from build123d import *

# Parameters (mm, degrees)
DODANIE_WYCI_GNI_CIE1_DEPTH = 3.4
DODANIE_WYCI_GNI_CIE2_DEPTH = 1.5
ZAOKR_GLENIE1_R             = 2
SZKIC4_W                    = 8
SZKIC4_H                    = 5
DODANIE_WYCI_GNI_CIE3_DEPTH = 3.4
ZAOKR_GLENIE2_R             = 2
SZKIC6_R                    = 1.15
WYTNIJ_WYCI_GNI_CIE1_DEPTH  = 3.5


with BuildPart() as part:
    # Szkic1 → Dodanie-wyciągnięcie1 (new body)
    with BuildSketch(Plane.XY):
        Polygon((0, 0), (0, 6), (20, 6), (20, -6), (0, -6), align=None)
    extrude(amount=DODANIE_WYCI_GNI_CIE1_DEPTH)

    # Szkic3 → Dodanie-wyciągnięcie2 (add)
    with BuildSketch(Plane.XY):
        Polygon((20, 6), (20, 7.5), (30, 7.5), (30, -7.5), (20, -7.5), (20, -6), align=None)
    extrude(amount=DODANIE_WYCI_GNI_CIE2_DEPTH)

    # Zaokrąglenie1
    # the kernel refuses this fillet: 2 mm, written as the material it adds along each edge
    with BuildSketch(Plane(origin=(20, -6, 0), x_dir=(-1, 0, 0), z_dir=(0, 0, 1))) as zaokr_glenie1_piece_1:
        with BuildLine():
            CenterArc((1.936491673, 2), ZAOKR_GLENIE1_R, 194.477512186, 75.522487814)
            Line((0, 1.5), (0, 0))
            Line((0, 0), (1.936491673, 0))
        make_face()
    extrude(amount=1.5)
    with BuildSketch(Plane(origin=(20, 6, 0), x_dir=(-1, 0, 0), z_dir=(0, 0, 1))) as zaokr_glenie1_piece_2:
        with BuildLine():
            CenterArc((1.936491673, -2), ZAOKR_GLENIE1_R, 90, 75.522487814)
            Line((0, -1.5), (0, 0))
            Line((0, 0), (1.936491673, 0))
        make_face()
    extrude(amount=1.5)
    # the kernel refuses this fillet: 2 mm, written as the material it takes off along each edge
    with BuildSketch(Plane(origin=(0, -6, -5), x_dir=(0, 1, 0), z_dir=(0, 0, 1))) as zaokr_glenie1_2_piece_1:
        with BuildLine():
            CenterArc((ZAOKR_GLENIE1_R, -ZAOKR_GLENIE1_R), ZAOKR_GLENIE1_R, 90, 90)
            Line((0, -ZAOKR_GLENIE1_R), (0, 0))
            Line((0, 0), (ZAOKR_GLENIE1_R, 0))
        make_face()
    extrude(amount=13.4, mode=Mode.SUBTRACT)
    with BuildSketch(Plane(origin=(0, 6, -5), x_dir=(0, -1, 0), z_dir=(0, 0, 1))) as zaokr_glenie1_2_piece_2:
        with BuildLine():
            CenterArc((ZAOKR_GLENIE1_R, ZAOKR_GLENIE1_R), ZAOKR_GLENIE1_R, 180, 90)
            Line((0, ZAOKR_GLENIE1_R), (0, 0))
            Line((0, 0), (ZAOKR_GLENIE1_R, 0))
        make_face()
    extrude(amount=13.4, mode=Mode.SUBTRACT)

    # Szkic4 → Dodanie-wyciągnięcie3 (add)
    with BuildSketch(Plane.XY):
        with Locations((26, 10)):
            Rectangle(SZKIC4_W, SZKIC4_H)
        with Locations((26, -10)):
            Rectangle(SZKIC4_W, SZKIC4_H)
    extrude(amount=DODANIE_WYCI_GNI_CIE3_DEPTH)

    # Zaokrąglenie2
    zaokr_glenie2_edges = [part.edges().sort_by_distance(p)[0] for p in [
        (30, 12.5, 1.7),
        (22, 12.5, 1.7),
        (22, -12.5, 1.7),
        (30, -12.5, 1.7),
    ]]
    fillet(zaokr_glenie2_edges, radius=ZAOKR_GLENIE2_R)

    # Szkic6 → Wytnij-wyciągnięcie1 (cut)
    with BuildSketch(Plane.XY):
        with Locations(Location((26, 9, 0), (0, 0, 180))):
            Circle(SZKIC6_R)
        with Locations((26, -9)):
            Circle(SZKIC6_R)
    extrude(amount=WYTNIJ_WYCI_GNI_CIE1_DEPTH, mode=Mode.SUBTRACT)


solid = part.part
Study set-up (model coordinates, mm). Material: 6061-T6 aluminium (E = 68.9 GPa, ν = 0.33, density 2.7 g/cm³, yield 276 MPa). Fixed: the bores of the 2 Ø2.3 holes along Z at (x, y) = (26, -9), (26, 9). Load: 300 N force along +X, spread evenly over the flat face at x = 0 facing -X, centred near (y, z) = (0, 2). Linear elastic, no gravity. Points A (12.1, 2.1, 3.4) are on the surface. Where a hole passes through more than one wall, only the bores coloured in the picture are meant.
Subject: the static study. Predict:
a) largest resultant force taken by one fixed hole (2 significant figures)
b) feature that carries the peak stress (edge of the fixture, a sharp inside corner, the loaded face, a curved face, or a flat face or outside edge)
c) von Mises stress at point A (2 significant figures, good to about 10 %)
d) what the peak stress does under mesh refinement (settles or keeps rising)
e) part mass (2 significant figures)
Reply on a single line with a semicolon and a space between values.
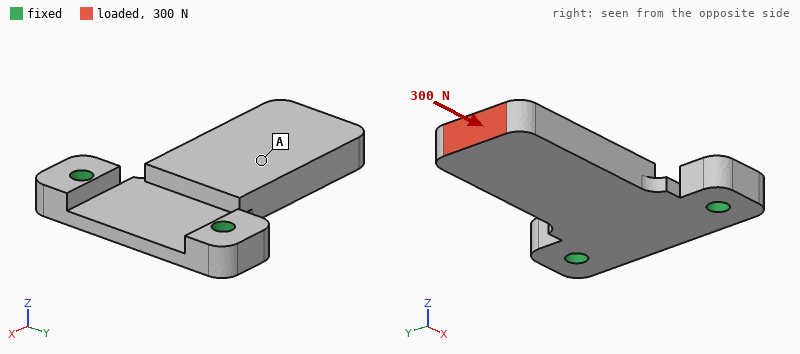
160 N; a sharp inside corner; 8.2 MPa; keeps rising; 3.4 g
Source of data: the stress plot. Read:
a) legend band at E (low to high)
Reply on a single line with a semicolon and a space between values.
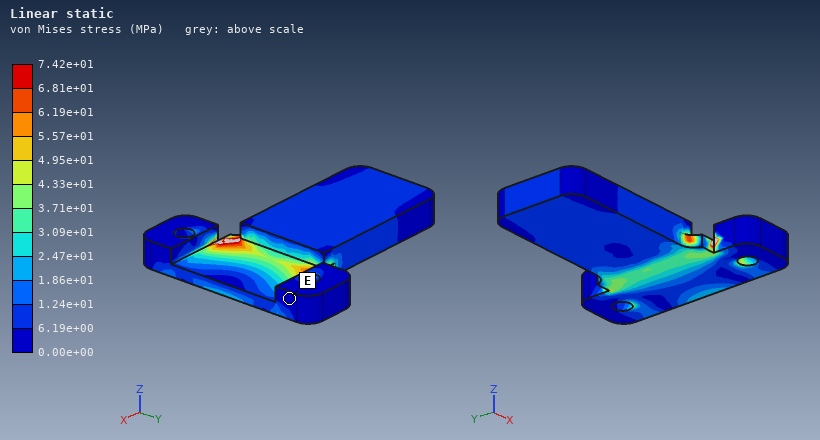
0.00e+00 to 6.19e+00 MPa
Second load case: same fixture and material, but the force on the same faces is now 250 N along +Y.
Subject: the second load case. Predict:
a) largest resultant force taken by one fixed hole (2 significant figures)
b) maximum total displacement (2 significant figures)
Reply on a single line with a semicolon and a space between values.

400 N; 62 µm
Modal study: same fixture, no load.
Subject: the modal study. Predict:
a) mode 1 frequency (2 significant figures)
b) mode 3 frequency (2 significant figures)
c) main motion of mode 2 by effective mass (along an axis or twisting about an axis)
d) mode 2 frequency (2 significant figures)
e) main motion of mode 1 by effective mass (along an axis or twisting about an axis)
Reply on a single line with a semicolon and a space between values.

1800 Hz; 13 kHz; along Y; 12 kHz; along Z
